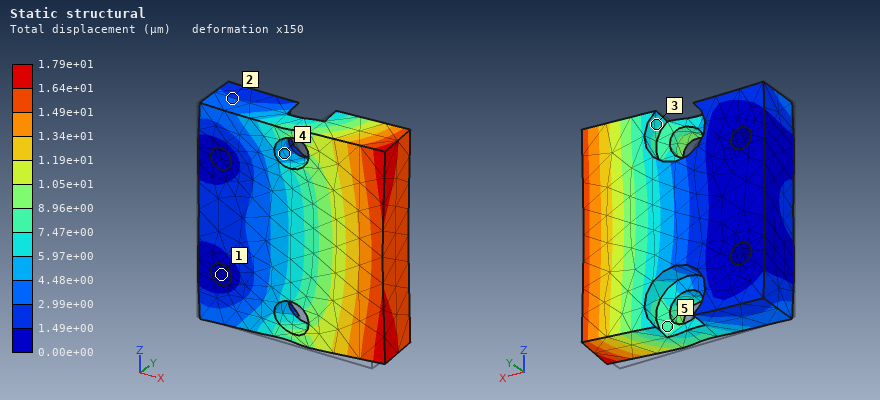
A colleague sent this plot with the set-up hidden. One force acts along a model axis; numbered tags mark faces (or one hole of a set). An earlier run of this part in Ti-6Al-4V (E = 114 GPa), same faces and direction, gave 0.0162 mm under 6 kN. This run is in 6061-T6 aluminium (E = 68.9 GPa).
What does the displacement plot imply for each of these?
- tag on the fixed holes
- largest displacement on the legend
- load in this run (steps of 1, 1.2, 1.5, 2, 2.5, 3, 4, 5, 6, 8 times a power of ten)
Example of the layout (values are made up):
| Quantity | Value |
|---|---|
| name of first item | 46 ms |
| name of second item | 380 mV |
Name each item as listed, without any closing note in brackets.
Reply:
| Quantity | Value |
|---|---|
| tag on the fixed holes | 1 |
| largest displacement on the legend | 1.79e+01 µm |
| load in this run | 4 kN |
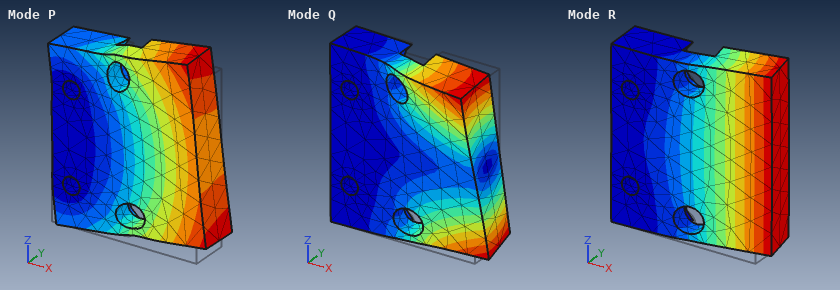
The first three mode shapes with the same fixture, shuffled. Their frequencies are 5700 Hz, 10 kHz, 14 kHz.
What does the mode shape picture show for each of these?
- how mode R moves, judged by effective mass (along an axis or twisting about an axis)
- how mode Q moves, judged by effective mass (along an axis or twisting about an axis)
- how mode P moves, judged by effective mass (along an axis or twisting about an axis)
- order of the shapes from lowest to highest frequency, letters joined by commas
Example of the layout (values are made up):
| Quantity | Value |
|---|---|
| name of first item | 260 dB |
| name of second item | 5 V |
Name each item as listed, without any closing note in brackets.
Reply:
| Quantity | Value |
|---|---|
| how mode R moves, judged by effective mass | along Y |
| how mode Q moves, judged by effective mass | twisting about X |
| how mode P moves, judged by effective mass | along Z |
| order of the shapes from lowest to highest frequency, letters joined by commas | R, Q, P |
